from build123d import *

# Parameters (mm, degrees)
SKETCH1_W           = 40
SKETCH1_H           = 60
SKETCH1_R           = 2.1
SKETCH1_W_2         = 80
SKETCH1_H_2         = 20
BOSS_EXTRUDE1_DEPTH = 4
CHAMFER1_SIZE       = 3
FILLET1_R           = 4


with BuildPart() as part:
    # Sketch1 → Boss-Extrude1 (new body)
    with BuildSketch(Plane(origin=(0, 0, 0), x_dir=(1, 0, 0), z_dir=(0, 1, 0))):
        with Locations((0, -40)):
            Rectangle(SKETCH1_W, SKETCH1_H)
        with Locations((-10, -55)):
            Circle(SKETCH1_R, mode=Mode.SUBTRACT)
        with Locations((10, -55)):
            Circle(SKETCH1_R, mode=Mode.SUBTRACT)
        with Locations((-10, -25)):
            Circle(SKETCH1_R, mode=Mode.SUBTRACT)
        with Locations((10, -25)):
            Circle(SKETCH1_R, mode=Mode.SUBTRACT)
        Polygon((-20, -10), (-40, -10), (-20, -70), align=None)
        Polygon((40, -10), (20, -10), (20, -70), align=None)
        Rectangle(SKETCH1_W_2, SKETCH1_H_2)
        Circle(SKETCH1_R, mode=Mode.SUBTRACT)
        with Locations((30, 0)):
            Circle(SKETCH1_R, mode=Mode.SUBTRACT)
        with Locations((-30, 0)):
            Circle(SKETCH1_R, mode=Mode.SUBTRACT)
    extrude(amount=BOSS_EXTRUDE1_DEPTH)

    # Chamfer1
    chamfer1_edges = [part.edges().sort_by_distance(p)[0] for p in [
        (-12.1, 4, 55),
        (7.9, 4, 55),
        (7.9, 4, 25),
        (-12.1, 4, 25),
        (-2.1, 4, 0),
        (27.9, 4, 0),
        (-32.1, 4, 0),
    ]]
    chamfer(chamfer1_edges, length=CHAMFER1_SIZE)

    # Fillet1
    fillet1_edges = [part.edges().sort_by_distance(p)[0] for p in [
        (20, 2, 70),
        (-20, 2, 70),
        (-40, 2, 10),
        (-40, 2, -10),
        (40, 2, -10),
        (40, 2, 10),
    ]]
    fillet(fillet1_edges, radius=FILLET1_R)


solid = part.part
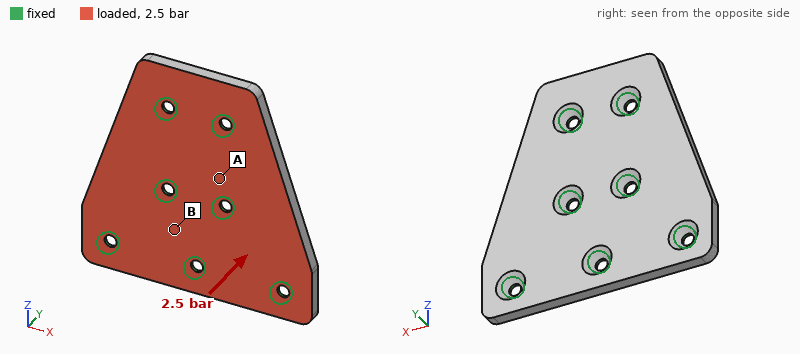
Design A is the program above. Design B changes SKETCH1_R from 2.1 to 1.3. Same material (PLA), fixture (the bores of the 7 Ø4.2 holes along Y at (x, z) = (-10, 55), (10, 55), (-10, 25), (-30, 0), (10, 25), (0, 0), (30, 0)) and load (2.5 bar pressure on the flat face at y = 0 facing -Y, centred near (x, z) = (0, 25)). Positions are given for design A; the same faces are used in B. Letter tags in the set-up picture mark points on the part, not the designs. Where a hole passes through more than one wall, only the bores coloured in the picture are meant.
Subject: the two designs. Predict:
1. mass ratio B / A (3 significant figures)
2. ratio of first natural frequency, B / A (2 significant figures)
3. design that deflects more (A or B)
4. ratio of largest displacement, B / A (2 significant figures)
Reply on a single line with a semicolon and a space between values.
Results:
1.02; 0.93; B; 1.1
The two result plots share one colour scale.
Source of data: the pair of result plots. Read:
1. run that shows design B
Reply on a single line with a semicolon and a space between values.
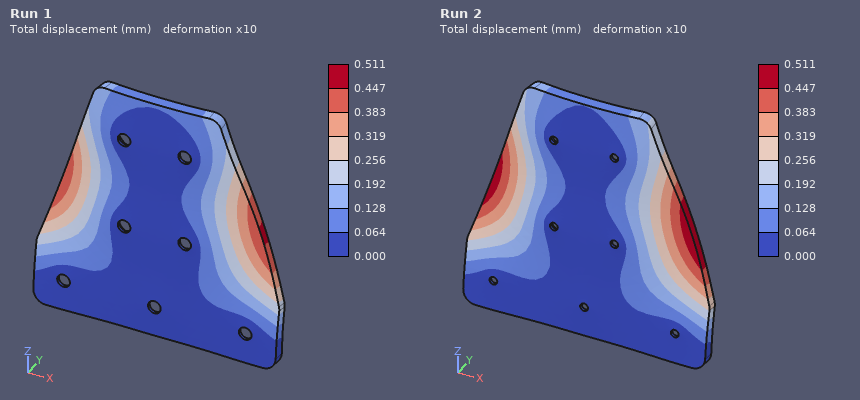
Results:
Run 2
